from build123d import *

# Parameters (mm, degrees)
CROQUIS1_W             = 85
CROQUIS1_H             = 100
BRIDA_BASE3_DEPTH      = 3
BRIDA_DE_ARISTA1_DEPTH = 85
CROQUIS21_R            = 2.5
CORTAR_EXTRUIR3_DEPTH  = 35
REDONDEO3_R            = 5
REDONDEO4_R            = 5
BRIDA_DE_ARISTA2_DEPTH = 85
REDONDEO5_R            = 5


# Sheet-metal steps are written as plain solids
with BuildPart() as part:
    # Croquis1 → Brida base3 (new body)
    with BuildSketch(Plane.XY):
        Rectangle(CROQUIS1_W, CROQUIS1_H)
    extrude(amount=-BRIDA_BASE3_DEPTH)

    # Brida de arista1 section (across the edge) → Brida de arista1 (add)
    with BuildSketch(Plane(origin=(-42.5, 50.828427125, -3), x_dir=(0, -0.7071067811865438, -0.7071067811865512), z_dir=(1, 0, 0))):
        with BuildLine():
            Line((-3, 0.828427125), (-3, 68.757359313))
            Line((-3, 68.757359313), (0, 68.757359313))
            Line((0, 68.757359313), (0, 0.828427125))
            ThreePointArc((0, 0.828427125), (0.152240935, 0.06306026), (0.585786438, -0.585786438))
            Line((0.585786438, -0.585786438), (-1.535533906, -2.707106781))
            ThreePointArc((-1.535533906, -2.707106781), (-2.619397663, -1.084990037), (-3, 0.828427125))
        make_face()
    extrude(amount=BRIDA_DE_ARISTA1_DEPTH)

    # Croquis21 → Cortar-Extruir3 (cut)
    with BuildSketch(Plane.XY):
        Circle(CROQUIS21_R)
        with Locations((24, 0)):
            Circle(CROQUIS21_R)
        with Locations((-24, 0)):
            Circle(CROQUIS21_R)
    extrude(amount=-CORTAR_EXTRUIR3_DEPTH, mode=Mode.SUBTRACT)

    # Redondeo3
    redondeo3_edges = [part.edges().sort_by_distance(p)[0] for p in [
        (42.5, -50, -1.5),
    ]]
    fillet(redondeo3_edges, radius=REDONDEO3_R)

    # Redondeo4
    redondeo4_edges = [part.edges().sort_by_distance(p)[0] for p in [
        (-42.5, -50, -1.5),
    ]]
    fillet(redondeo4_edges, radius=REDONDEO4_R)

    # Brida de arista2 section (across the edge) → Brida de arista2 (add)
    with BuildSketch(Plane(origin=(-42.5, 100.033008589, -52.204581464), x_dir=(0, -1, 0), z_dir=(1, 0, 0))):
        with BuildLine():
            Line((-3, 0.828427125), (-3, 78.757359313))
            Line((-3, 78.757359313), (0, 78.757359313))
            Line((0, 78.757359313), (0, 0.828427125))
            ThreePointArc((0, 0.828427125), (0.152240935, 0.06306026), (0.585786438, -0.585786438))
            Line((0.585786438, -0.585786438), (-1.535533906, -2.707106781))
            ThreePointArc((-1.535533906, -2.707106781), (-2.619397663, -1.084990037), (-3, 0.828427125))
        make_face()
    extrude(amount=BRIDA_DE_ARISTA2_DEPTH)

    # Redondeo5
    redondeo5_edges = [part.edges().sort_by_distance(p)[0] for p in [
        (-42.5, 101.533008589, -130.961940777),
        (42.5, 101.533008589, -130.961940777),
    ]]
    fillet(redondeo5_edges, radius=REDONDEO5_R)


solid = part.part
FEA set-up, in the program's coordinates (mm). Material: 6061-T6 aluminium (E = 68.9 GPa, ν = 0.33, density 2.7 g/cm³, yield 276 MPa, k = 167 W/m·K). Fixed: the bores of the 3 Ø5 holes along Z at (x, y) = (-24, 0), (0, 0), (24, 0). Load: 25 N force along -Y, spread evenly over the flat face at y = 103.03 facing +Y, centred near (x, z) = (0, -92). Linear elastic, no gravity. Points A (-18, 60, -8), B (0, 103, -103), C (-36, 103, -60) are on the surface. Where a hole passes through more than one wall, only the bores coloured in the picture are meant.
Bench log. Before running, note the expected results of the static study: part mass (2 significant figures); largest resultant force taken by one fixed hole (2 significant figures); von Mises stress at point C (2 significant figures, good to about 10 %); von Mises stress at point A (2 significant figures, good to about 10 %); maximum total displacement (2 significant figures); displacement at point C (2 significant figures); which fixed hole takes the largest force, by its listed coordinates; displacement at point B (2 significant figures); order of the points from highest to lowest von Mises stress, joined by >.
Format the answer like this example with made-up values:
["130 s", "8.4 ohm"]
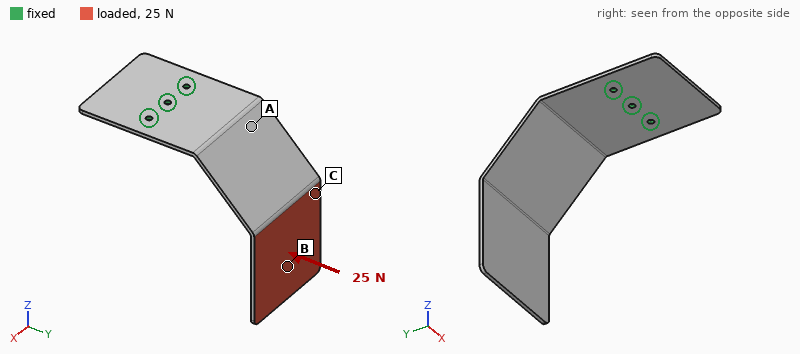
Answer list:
["170 g", "15 N", "5.5 MPa", "14 MPa", "2.2 mm", "1.2 mm", "(0, 0)", "1.8 mm", "A > C > B"]
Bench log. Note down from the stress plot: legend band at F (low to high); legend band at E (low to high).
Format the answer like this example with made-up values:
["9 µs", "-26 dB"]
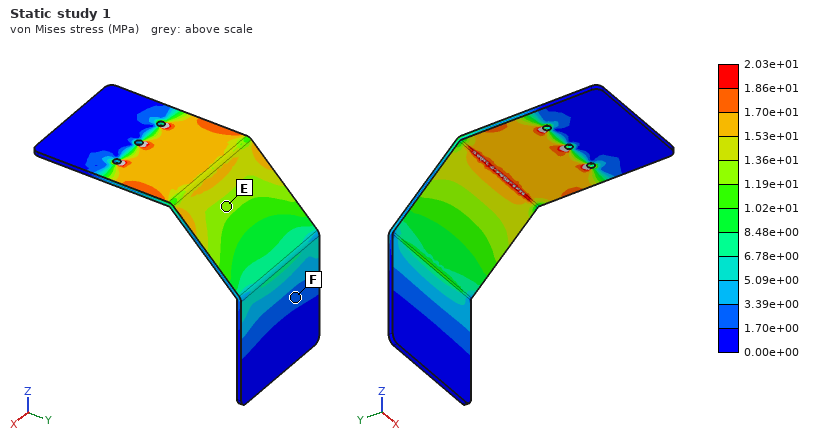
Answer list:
["1.70e+00 to 3.39e+00 MPa", "1.19e+01 to 1.36e+01 MPa"]
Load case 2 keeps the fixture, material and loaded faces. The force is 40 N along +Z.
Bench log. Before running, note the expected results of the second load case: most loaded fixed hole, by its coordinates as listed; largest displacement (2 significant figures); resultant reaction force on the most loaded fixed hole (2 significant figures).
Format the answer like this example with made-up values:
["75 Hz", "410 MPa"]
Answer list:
["(0, 0)", "2.3 mm", "24 N"]
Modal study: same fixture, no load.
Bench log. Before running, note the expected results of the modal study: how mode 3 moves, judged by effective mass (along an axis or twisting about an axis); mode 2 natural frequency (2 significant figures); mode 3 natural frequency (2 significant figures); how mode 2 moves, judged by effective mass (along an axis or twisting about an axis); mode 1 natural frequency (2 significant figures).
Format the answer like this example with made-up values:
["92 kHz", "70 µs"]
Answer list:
["along Z", "150 Hz", "280 Hz", "along X", "71 Hz"]
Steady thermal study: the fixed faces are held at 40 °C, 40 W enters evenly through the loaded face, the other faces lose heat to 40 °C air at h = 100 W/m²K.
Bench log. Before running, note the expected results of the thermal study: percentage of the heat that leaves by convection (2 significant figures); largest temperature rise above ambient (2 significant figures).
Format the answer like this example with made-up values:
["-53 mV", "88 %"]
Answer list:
["93 %", "35 K"]
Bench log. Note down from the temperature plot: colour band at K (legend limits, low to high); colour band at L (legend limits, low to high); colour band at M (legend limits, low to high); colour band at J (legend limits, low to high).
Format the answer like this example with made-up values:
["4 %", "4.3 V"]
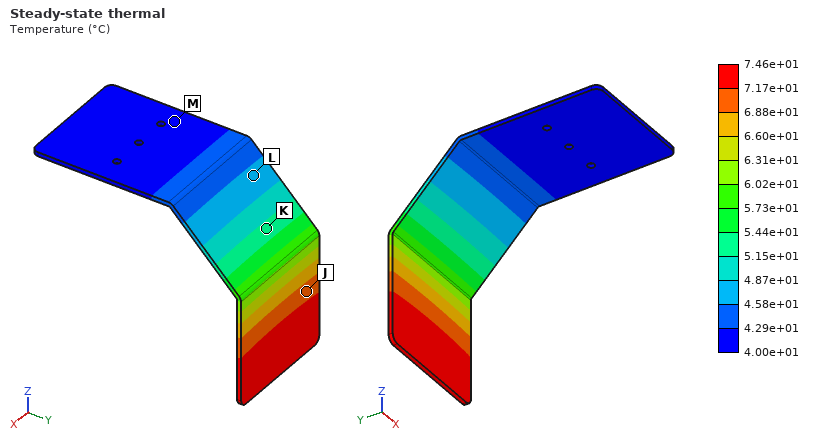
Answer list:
["5.15e+01 to 5.44e+01 °C", "4.58e+01 to 4.87e+01 °C", "4.00e+01 to 4.29e+01 °C", "6.88e+01 to 7.17e+01 °C"]
